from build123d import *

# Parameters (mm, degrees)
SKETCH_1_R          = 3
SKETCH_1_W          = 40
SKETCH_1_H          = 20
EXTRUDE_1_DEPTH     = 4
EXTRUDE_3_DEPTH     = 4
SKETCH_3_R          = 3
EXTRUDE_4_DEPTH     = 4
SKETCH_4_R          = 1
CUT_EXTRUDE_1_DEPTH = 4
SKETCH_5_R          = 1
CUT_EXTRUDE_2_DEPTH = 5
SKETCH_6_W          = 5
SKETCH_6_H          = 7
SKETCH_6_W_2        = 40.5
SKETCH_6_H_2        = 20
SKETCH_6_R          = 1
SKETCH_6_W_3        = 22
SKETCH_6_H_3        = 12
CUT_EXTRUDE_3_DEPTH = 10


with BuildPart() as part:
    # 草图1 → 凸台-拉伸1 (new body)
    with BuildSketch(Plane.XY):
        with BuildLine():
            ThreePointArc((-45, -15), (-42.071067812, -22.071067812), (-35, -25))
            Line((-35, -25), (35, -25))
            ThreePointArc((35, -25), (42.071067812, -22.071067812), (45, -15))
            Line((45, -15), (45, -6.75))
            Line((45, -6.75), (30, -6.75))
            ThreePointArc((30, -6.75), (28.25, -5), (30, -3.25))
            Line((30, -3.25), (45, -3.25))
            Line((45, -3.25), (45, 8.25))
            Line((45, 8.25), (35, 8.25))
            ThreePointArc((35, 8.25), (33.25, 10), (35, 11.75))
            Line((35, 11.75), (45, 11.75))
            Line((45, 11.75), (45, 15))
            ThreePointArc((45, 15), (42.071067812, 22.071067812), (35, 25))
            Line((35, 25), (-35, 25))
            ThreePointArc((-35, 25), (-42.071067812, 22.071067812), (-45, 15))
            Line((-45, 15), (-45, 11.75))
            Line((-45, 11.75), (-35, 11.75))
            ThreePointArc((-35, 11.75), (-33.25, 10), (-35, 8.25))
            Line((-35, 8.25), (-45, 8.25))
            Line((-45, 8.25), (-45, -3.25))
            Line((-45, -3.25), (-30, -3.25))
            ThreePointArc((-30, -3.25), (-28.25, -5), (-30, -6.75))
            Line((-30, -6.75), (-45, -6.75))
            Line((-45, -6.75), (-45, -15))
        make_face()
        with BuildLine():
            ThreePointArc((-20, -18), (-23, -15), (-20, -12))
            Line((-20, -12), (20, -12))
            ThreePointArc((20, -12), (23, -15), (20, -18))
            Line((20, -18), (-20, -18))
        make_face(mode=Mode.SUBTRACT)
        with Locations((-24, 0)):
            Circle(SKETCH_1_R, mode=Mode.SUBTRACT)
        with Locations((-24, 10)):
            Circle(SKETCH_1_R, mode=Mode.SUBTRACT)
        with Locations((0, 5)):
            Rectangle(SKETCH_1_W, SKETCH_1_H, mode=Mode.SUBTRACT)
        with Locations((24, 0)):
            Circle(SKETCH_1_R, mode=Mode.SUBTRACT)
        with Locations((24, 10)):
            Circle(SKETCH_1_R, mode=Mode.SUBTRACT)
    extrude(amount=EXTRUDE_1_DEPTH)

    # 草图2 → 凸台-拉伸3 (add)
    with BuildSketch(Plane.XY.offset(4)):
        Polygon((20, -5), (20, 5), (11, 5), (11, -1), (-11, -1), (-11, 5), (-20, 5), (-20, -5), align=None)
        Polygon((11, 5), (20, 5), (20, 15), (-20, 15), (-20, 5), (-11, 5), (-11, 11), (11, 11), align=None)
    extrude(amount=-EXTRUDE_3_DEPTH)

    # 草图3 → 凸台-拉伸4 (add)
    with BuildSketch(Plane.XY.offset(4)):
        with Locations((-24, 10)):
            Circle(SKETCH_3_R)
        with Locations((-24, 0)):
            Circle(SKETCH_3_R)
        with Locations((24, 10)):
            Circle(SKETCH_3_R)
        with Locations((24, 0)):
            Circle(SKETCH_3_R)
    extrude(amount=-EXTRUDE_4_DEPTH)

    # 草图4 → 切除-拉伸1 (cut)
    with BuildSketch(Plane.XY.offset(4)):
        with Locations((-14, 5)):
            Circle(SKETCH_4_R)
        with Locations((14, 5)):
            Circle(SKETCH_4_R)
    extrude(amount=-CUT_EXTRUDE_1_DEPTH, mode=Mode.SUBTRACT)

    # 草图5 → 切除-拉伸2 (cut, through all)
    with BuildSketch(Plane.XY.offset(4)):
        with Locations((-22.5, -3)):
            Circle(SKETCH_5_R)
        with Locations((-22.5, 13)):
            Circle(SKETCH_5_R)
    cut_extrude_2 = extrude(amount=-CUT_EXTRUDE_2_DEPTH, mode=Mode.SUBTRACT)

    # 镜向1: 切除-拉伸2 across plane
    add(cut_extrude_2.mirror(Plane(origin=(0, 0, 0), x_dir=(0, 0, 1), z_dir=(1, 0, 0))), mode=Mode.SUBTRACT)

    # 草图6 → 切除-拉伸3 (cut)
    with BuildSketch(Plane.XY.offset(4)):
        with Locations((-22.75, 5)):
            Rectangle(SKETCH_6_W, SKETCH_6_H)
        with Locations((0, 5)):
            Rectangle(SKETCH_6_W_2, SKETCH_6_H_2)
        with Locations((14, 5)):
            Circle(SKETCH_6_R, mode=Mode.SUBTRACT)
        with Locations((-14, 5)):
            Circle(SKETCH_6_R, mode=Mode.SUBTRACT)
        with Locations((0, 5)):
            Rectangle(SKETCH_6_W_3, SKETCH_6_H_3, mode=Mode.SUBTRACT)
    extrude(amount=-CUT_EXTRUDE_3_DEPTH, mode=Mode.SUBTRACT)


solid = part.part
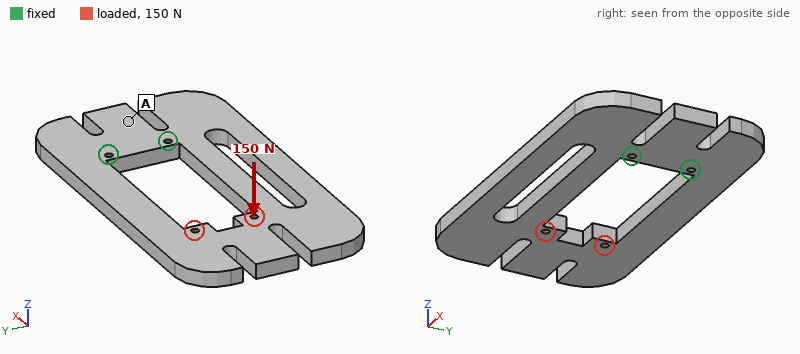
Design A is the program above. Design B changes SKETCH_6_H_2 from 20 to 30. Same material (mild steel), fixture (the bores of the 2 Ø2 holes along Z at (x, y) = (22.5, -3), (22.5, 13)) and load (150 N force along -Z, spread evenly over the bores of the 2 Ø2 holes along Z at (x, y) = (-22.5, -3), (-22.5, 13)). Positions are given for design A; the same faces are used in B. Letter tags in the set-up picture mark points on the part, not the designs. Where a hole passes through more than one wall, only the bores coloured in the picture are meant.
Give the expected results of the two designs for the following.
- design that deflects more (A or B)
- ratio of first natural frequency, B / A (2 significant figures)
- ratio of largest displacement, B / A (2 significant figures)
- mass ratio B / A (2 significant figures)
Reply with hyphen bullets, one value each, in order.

- B
- 0.76
- 1.9
- 0.87
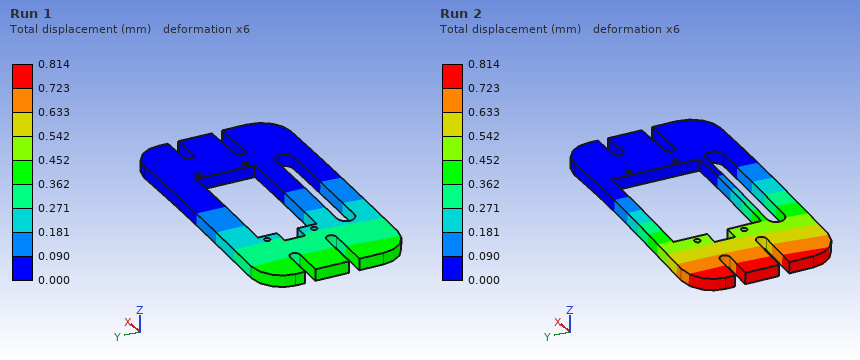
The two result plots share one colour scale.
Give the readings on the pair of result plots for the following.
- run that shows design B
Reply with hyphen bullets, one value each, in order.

- Run 2
